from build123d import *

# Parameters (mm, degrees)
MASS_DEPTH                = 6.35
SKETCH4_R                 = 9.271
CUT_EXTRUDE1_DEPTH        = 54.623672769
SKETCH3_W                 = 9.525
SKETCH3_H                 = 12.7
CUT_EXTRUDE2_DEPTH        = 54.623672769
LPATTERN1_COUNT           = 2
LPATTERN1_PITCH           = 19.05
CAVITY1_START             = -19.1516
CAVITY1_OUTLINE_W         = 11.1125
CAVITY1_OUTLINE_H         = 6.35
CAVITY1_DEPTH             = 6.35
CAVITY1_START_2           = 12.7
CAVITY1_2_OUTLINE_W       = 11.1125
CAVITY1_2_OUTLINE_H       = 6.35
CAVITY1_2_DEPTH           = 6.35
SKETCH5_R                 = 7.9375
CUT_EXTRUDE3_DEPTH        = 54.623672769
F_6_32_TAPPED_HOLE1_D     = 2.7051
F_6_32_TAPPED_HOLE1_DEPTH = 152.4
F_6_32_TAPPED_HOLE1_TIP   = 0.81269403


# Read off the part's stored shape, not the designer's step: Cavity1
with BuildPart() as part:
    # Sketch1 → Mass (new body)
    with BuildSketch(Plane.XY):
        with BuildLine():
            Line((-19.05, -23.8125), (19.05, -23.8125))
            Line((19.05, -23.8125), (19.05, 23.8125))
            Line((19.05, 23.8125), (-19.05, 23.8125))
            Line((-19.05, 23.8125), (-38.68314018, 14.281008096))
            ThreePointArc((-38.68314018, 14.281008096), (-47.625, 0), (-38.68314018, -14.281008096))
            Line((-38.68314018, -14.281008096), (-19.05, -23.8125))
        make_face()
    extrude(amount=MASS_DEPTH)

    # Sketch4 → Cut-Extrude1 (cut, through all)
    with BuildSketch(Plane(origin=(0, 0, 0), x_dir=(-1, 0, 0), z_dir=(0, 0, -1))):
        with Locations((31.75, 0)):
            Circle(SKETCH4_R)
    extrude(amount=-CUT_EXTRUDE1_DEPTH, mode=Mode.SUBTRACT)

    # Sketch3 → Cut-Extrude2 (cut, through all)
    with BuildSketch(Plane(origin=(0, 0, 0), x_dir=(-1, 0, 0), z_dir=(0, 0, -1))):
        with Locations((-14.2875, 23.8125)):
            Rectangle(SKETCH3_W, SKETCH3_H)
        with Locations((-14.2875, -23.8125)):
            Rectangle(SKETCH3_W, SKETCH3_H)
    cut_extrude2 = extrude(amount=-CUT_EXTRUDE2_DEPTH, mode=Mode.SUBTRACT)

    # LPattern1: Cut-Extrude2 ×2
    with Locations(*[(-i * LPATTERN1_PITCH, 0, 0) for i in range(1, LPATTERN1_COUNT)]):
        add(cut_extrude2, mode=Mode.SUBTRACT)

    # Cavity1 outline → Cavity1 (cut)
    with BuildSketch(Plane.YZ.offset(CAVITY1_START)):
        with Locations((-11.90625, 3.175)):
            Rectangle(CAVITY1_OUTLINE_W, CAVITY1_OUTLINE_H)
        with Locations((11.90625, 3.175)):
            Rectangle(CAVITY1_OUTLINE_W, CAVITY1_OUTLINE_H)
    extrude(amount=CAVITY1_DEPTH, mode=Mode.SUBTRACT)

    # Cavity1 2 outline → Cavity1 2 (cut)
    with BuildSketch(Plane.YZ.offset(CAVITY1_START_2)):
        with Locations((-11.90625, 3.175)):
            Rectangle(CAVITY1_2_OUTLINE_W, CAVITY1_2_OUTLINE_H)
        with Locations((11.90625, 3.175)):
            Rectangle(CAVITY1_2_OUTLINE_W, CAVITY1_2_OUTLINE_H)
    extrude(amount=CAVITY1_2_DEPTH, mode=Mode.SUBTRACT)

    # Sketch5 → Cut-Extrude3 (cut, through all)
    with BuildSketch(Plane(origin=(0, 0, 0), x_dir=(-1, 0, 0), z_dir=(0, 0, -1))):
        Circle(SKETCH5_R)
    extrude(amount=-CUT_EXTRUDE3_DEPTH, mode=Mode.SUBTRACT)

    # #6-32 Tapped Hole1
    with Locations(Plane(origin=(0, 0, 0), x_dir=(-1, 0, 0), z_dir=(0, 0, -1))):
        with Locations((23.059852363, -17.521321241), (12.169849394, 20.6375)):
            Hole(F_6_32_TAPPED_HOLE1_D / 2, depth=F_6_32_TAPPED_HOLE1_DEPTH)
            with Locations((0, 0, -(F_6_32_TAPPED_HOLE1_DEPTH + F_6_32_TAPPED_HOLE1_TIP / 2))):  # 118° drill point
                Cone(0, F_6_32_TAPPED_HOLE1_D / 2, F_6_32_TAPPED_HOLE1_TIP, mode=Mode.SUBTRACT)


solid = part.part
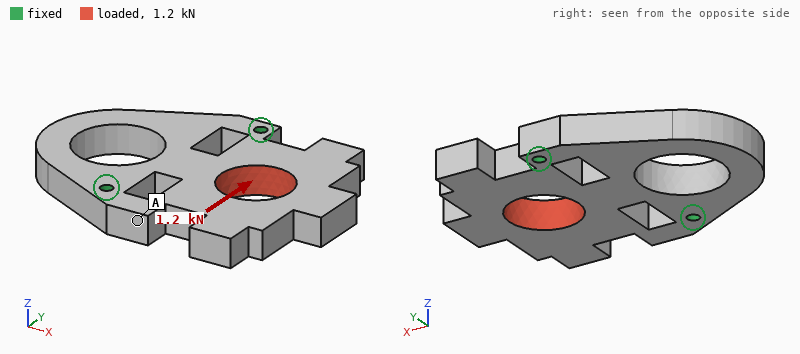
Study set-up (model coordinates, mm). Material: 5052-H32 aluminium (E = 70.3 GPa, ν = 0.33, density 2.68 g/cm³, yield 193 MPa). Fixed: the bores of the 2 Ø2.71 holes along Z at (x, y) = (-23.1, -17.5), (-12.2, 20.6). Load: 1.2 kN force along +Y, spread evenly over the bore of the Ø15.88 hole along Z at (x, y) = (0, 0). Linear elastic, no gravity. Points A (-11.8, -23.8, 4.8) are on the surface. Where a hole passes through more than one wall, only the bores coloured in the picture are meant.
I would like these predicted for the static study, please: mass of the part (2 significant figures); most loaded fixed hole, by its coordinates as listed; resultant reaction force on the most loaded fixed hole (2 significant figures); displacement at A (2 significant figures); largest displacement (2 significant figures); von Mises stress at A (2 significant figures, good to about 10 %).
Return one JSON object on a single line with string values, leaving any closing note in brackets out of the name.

{"mass of the part": "30 g", "most loaded fixed hole, by its coordinates as listed": "(-12.2, 20.6)", "resultant reaction force on the most loaded fixed hole": "920 N", "displacement at A": "6.1 µm", "largest displacement": "19 µm", "von Mises stress at A": "4.7 MPa"}
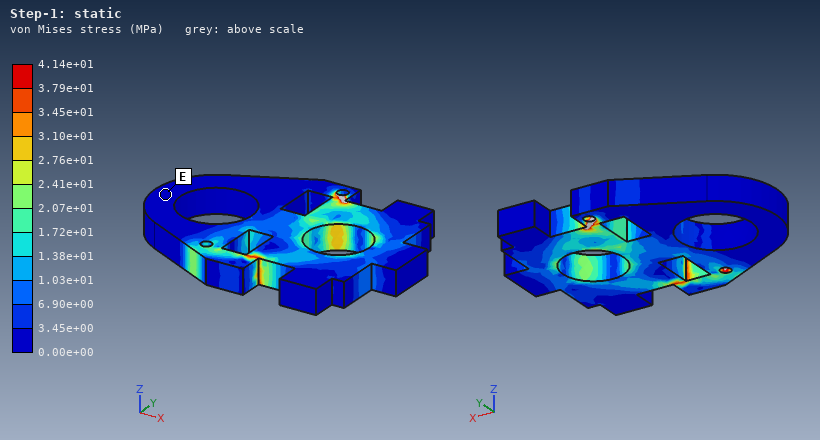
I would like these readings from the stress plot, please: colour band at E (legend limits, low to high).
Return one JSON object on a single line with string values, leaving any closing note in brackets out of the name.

{"colour band at E": "0.00e+00 to 3.45e+00 MPa"}
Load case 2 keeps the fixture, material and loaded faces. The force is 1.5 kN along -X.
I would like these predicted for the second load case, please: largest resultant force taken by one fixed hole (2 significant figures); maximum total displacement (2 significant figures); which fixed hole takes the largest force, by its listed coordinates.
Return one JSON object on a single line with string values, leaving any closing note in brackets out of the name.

{"largest resultant force taken by one fixed hole": "870 N", "maximum total displacement": "10 µm", "which fixed hole takes the largest force, by its listed coordinates": "(-23.1, -17.5)"}
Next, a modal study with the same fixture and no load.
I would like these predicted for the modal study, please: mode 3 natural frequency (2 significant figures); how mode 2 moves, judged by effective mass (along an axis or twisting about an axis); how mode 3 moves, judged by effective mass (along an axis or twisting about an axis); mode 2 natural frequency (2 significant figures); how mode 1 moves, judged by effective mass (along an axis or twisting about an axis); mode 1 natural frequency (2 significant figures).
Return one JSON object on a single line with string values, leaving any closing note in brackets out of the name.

{"mode 3 natural frequency": "6800 Hz", "how mode 2 moves, judged by effective mass": "along Z", "how mode 3 moves, judged by effective mass": "twisting about X", "mode 2 natural frequency": "5600 Hz", "how mode 1 moves, judged by effective mass": "along Z", "mode 1 natural frequency": "2700 Hz"}
